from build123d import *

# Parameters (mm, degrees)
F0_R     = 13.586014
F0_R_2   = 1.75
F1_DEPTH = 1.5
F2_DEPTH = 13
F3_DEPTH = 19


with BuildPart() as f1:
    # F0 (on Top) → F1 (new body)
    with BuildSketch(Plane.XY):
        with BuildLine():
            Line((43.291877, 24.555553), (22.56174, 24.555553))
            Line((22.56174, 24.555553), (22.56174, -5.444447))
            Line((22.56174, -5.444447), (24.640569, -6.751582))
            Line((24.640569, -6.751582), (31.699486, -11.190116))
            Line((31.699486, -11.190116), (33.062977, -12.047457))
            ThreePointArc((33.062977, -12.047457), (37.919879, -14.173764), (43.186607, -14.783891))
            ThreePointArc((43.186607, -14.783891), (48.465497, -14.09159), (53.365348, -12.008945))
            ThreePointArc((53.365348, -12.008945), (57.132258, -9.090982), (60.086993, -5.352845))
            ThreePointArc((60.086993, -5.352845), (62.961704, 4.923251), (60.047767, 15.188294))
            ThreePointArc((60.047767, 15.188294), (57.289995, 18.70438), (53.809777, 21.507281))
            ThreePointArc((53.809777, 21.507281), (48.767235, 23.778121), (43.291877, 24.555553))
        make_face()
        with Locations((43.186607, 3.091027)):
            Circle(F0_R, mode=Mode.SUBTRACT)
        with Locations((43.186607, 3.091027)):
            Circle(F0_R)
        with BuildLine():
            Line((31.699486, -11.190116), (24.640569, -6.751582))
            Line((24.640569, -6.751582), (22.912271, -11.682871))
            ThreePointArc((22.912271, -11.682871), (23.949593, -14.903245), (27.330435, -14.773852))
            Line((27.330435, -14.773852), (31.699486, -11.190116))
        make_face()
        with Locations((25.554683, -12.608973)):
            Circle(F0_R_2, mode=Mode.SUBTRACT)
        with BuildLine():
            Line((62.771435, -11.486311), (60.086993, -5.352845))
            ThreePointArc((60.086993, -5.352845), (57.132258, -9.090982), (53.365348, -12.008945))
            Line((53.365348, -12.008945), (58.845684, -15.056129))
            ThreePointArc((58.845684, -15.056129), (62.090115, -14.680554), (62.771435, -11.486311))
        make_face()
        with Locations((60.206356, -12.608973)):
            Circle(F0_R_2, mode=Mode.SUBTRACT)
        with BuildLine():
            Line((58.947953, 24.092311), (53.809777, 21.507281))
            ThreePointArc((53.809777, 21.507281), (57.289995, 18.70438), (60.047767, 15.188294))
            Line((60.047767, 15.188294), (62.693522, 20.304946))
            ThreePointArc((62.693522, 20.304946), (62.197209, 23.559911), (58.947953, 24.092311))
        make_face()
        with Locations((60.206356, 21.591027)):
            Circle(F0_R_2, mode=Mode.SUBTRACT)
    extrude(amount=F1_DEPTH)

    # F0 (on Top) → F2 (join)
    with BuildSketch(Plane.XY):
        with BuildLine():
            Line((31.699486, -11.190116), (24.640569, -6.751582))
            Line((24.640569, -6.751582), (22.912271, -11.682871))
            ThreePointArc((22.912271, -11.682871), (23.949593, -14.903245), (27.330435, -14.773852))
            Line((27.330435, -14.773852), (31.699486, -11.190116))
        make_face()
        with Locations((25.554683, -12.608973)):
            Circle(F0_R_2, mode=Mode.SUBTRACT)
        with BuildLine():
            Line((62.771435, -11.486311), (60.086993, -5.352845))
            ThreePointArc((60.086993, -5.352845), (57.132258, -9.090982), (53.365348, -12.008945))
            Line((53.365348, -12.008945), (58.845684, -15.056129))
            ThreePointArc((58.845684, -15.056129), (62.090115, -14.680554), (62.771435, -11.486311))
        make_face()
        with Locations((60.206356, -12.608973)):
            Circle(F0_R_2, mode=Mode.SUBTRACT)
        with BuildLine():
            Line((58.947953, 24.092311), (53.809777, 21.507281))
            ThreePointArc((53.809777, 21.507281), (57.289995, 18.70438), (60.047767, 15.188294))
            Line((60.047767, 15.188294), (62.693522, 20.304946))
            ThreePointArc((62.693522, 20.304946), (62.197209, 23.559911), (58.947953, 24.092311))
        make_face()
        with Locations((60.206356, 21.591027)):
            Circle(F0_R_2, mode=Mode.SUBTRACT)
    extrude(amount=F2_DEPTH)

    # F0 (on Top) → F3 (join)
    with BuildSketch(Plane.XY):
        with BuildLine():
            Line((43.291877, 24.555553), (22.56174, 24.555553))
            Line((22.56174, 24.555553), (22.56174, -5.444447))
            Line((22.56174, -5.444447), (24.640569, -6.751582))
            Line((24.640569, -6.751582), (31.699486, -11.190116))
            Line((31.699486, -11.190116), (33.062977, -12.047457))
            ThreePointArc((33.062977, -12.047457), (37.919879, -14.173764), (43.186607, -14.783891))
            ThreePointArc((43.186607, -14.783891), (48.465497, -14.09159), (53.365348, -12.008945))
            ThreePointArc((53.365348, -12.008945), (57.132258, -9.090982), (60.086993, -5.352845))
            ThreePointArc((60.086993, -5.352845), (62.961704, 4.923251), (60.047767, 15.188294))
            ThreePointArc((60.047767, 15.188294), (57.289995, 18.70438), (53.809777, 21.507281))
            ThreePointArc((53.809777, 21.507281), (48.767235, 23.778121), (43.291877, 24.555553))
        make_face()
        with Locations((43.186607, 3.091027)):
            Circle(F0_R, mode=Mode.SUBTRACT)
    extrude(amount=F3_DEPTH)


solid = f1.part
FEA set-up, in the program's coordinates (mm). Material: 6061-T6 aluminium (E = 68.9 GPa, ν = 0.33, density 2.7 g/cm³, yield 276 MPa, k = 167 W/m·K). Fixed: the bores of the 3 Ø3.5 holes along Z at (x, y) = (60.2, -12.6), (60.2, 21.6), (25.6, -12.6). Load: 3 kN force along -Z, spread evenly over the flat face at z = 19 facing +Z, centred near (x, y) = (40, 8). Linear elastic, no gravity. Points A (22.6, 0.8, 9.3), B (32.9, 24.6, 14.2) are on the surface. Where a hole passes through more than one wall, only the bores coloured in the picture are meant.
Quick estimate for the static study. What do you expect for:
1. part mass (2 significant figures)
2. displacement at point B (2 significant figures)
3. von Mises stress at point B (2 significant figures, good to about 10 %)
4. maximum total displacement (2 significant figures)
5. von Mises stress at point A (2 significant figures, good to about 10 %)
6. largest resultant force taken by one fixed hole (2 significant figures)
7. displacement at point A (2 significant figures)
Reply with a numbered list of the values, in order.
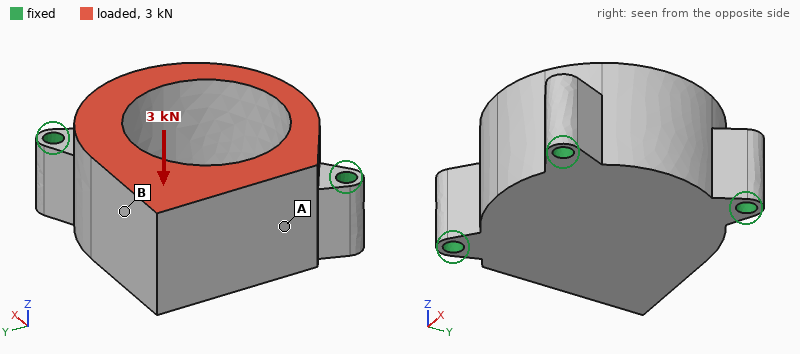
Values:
1. 46 g
2. 33 µm
3. 9.5 MPa
4. 44 µm
5. 22 MPa
6. 1.5 kN
7. 16 µm
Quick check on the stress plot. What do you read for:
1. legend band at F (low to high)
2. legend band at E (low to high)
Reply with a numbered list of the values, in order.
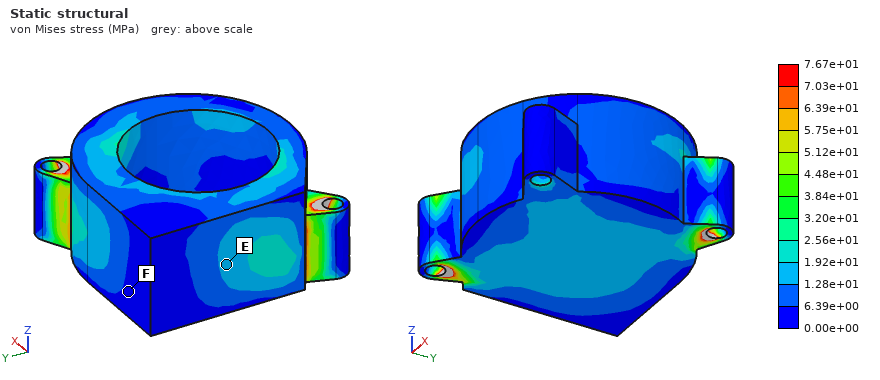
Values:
1. 0.00e+00 to 6.39e+00 MPa
2. 1.28e+01 to 1.92e+01 MPa
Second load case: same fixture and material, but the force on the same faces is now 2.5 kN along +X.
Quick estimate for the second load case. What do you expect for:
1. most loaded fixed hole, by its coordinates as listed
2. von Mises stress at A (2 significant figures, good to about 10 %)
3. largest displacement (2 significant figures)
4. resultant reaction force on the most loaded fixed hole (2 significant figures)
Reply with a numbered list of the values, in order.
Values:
1. (60.2, 21.6)
2. 16 MPa
3. 30 µm
4. 1.6 kN
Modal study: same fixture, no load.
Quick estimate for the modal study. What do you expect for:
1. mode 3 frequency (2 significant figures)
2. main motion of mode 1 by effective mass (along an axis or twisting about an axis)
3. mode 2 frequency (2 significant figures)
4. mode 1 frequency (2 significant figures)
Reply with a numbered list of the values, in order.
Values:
1. 19 kHz
2. along Z
3. 18 kHz
4. 8200 Hz
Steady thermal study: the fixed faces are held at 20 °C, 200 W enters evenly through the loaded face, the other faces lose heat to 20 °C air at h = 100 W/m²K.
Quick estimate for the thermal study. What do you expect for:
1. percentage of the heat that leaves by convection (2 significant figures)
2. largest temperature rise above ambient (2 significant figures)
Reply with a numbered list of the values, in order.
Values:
1. 9.3 %
2. 64 K
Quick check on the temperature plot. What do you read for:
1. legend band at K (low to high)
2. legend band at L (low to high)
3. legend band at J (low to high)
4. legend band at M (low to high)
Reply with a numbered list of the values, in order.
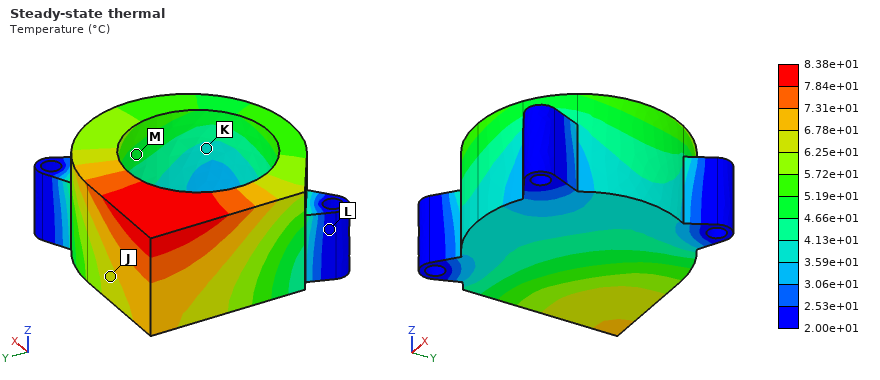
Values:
1. 3.59e+01 to 4.13e+01 °C
2. 2.00e+01 to 2.53e+01 °C
3. 6.25e+01 to 6.78e+01 °C
4. 4.66e+01 to 5.19e+01 °C
